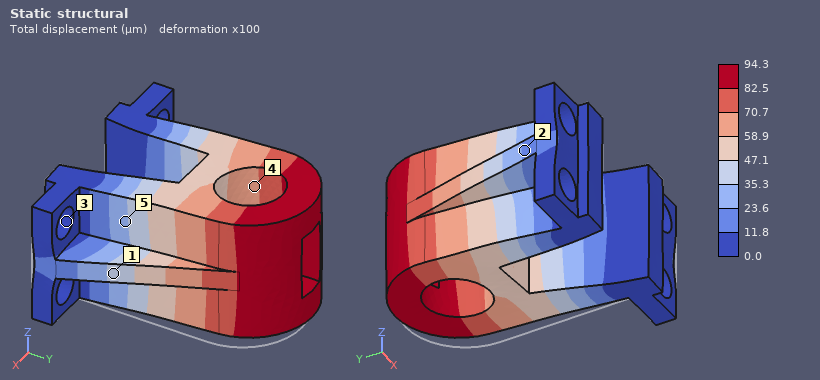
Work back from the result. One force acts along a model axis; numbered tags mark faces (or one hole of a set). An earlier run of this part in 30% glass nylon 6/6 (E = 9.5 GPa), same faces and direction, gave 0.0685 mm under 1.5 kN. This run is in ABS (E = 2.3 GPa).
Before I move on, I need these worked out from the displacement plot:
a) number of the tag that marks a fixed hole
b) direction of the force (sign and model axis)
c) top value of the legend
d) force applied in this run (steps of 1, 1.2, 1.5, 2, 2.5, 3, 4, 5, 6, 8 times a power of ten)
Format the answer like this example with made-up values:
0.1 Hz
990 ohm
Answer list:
3
-X
94.3 µm
500 N
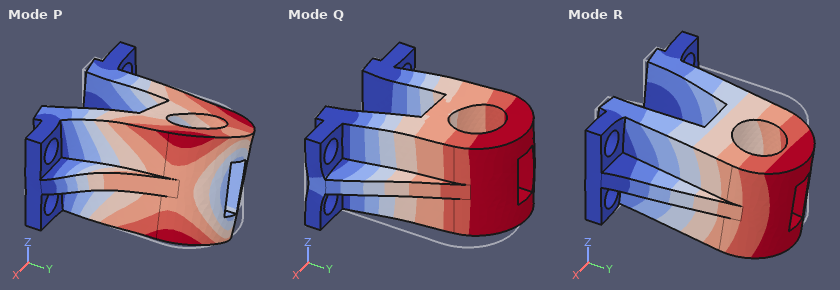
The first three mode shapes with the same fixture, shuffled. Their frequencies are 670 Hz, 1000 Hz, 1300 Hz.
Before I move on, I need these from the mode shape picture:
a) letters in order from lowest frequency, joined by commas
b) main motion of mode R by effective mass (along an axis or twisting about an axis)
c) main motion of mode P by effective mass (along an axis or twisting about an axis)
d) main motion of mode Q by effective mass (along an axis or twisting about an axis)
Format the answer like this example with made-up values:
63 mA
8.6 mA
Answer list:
R, Q, P
along Z
twisting about Y
along X
